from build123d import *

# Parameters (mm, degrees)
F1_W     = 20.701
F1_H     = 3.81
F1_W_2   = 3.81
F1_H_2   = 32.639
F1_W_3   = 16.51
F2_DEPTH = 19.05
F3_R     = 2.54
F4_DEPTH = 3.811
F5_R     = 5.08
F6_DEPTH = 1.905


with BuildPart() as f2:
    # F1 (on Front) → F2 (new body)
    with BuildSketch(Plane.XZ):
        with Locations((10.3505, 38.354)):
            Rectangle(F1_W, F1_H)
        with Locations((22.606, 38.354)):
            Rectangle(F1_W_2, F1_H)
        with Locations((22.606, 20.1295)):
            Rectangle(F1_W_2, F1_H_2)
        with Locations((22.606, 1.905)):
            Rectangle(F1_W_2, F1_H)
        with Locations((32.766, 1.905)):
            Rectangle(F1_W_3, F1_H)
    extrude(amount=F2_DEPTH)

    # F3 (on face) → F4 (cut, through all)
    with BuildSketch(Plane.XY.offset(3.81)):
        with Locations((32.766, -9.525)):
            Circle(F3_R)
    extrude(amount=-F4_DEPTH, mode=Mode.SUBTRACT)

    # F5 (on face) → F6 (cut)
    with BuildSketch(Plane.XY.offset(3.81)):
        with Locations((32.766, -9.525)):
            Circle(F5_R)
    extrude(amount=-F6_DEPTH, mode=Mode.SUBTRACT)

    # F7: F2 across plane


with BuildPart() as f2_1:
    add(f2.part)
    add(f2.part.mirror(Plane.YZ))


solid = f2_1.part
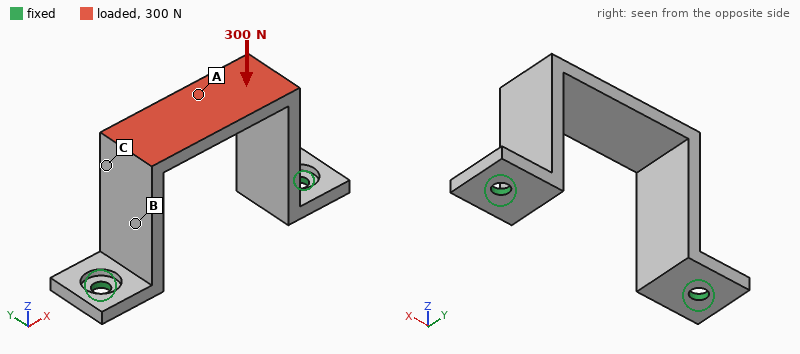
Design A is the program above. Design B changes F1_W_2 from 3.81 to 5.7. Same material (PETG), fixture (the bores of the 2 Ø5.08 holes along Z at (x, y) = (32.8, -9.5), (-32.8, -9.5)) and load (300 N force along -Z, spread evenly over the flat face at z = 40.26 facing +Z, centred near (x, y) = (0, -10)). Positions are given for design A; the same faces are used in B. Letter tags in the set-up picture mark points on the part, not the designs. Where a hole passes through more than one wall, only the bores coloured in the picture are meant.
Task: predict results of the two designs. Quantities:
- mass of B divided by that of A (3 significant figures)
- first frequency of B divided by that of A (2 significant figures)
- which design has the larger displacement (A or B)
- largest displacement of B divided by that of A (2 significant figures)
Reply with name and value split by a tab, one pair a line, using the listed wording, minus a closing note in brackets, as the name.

mass of B divided by that of A	1.24
first frequency of B divided by that of A	0.99
which design has the larger displacement	A
largest displacement of B divided by that of A	0.62
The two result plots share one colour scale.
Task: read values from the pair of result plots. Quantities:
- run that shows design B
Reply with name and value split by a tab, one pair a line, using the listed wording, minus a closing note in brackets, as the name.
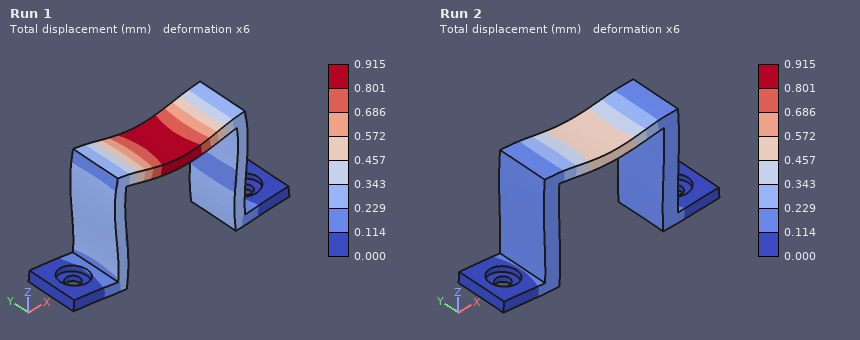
run that shows design B	Run 2
